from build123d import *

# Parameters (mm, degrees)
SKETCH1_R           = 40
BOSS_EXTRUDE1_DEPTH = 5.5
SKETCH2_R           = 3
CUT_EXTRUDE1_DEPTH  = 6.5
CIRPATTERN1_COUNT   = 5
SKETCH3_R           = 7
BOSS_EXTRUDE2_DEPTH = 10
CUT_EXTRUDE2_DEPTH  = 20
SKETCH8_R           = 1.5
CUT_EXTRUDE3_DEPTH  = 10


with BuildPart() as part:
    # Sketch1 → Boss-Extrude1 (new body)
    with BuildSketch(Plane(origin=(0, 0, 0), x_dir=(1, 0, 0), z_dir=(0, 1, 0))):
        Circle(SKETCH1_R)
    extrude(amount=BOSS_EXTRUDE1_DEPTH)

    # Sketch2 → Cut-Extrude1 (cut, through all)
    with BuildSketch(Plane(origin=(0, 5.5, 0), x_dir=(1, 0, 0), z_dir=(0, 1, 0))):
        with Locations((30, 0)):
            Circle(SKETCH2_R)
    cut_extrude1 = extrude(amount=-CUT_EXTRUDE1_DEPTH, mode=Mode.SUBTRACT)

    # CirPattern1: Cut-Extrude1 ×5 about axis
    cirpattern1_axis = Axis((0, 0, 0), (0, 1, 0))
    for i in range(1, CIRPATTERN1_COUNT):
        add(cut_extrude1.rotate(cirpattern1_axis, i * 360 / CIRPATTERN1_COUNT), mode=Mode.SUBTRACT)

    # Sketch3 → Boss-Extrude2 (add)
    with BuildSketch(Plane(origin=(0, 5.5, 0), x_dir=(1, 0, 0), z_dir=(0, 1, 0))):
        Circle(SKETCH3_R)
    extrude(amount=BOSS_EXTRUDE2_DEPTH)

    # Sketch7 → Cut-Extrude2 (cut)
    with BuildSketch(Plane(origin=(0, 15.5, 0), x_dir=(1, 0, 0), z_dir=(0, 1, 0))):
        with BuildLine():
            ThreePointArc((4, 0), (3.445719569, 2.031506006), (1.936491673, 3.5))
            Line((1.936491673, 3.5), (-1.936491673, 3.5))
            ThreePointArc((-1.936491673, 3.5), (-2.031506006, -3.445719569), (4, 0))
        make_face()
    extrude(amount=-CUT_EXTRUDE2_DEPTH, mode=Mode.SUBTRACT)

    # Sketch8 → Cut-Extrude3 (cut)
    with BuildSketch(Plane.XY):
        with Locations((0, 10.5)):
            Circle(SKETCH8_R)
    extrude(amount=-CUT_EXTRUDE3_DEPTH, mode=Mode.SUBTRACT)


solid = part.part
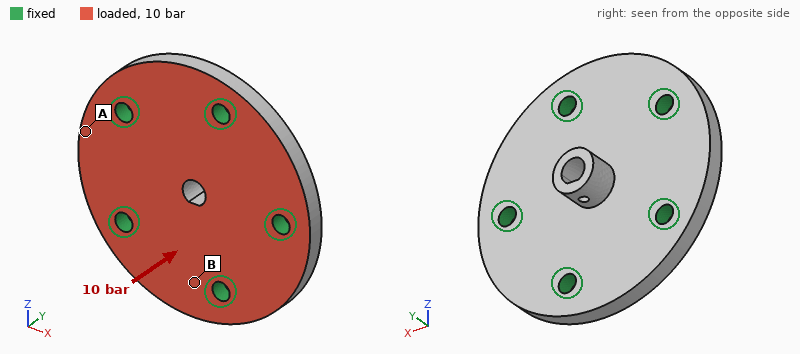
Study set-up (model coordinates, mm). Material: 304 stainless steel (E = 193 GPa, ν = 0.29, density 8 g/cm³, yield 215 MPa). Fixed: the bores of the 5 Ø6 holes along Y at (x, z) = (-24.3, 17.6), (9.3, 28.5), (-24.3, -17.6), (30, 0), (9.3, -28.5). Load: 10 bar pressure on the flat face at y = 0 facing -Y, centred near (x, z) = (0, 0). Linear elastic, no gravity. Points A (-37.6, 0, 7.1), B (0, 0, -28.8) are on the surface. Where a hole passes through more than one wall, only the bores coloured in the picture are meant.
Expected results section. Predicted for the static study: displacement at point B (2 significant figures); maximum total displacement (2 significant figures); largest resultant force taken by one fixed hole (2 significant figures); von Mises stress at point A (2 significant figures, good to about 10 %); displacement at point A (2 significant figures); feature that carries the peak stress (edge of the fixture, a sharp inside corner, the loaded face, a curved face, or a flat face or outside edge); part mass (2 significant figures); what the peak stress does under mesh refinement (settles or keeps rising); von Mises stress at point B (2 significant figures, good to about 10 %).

1.3 µm
4.7 µm
970 N
5.3 MPa
2.4 µm
edge of the fixture
220 g
keeps rising
9.9 MPa
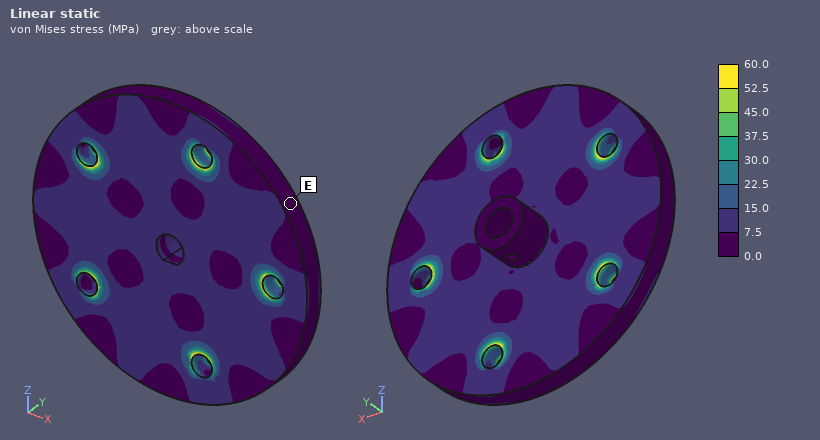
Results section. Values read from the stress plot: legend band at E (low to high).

0.0 to 7.5 MPa
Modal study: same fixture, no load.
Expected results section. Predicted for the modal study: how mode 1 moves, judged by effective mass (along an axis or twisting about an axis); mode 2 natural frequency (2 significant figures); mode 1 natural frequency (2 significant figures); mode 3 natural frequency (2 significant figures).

along Y
15 kHz
11 kHz
15 kHz
